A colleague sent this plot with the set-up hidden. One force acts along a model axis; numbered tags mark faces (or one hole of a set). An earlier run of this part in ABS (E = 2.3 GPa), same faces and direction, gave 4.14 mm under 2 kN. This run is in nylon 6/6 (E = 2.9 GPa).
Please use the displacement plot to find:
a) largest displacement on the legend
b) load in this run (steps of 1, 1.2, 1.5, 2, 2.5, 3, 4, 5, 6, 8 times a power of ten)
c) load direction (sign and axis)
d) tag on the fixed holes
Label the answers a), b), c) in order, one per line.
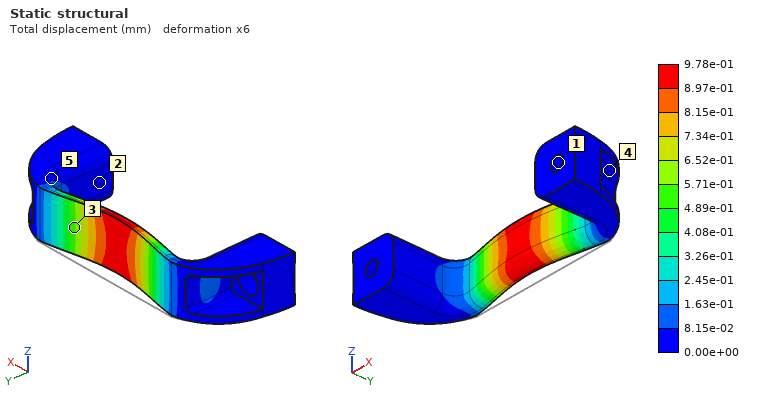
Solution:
a) 9.78e-01 mm
b) 600 N
c) -Y
d) 1
